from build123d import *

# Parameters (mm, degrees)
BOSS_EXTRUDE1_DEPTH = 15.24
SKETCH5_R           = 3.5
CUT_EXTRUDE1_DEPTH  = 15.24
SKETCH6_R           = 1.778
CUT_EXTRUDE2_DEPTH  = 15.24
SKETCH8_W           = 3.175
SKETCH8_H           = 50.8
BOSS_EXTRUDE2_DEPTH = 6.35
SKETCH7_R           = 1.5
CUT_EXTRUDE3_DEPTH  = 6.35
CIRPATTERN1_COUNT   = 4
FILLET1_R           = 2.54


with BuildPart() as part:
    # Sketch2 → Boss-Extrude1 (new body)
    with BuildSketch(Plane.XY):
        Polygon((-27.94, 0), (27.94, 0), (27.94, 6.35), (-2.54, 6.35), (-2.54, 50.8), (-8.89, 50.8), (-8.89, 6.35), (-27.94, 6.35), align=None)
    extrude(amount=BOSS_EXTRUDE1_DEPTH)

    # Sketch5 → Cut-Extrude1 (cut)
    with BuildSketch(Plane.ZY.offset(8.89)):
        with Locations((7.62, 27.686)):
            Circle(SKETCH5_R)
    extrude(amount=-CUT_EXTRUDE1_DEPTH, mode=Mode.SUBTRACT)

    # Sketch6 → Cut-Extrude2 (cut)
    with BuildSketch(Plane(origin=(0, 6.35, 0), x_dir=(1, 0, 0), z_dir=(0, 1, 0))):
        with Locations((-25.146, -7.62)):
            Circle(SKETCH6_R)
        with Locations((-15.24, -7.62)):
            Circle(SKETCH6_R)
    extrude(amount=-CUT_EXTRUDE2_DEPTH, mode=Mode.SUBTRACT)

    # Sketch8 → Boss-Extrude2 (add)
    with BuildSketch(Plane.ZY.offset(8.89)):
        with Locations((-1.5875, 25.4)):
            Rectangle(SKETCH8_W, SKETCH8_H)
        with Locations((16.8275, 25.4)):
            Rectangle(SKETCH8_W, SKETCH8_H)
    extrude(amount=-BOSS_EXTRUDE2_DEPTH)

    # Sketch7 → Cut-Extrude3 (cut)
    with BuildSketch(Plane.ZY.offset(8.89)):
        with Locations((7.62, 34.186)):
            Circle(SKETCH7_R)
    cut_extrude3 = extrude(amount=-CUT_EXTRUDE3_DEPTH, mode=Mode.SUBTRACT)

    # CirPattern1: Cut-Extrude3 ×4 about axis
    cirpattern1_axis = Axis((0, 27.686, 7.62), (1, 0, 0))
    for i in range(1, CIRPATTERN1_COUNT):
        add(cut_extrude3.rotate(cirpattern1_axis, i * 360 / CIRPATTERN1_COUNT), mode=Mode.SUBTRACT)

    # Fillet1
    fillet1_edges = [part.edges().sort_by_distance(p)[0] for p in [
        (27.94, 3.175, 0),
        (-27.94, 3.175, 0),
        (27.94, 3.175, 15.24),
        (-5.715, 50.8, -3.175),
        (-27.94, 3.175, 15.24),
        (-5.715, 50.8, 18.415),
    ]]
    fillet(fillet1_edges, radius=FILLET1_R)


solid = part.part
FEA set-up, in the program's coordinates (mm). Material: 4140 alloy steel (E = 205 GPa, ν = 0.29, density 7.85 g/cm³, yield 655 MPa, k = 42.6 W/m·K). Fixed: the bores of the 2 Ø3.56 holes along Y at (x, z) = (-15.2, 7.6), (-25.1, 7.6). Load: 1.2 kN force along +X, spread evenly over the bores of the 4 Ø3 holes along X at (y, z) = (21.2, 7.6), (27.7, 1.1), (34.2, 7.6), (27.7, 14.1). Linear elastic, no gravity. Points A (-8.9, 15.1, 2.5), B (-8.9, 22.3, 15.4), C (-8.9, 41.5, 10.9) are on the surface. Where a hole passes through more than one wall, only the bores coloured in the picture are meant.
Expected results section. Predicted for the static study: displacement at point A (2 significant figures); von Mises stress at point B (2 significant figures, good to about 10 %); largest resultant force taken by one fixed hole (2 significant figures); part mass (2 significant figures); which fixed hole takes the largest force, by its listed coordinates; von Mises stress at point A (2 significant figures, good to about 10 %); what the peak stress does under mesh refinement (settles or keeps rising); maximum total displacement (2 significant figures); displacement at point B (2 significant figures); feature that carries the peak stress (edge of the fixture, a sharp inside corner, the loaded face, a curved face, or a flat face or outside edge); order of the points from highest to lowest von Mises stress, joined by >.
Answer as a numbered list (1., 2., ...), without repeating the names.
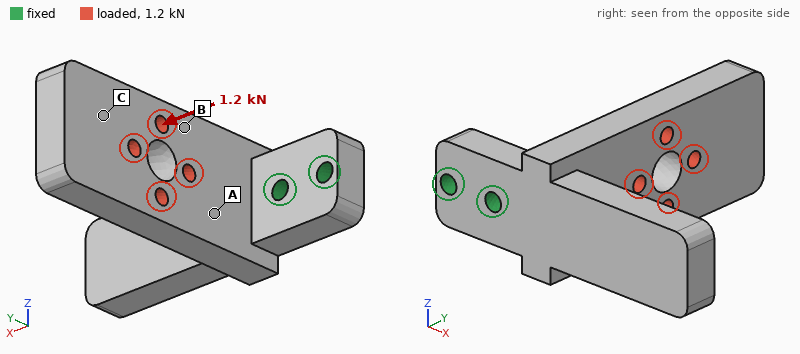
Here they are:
1. 0.058 mm
2. 57 MPa
3. 1.3 kN
4. 88 g
5. (-15.2, 7.6)
6. 100 MPa
7. keeps rising
8. 0.32 mm
9. 0.11 mm
10. edge of the fixture
11. A > B > C
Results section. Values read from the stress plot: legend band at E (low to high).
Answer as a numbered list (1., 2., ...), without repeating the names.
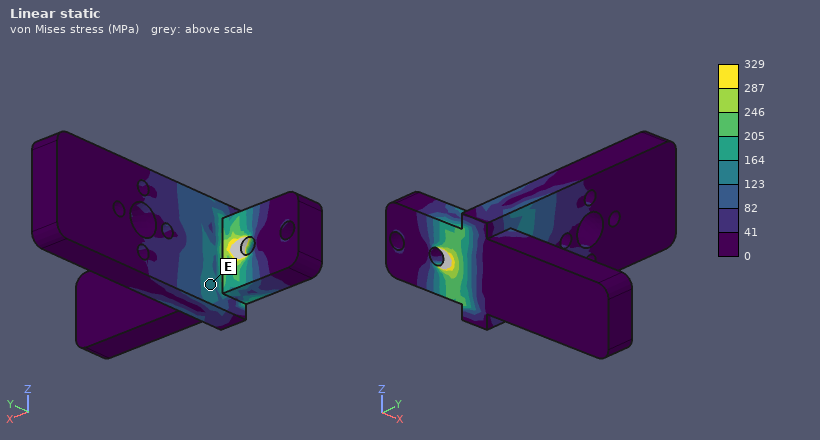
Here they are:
1. 123 to 164 MPa
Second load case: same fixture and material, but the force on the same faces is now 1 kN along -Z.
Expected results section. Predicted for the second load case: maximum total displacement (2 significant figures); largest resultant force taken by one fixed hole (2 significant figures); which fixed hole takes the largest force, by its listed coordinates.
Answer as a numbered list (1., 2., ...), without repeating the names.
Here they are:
1. 0.12 mm
2. 1.5 kN
3. (-15.2, 7.6)
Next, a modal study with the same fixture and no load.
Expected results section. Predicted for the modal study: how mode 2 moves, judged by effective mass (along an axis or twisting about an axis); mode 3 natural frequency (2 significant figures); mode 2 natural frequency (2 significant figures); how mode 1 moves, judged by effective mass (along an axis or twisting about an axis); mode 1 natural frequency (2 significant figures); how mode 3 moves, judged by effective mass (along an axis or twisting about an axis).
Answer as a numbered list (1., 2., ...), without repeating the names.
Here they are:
1. along Z
2. 3800 Hz
3. 2500 Hz
4. along X
5. 1600 Hz
6. along Y
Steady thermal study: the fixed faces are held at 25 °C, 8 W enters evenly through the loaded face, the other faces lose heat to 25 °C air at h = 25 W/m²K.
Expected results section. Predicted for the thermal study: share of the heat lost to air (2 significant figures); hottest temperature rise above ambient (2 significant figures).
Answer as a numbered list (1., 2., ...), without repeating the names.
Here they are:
1. 32 %
2. 40 K
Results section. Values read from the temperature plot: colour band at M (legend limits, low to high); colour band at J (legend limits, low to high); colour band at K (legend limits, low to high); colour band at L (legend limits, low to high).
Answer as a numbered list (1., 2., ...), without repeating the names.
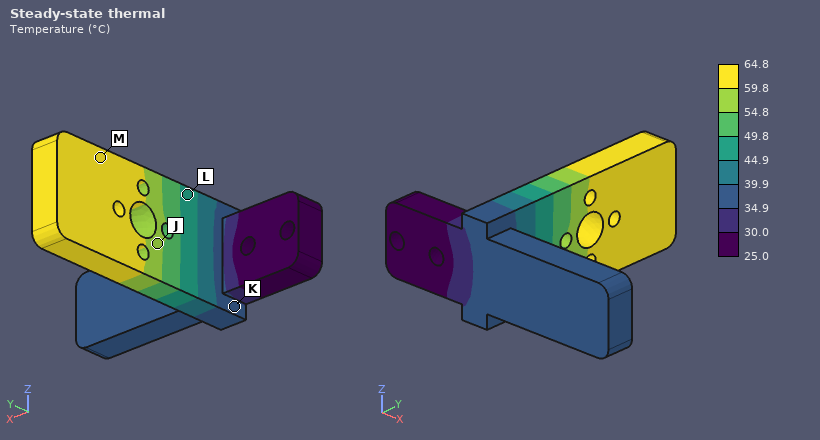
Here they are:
1. 59.8 to 64.8 °C
2. 54.8 to 59.8 °C
3. 34.9 to 39.9 °C
4. 44.9 to 49.8 °C
